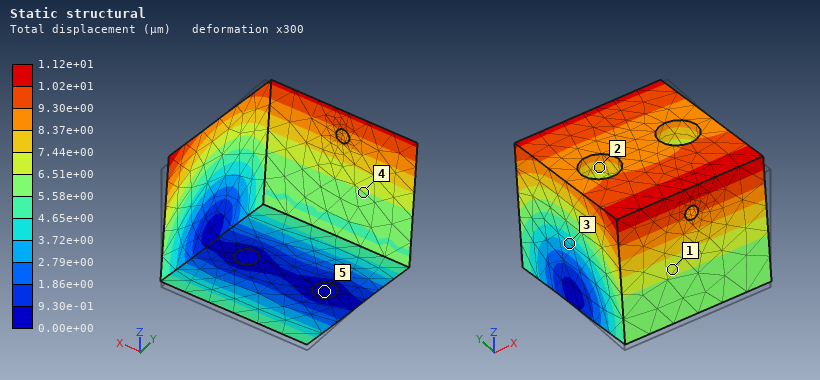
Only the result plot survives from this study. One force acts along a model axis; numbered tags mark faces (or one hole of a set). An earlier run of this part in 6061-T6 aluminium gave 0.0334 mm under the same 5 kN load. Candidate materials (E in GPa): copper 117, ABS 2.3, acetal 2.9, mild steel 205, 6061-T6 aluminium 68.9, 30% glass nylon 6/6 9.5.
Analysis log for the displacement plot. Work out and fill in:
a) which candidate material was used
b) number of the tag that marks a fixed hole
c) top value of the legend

mild steel
5
1.12e+01 µm
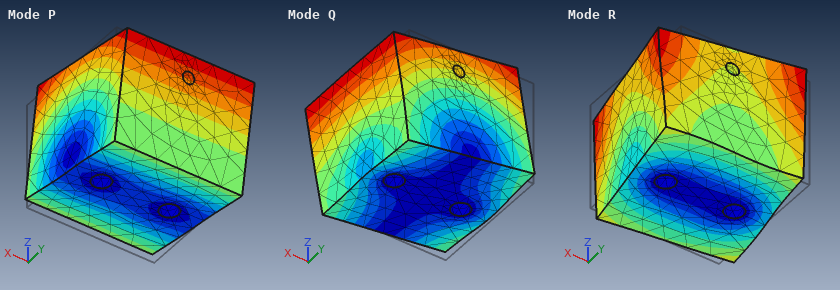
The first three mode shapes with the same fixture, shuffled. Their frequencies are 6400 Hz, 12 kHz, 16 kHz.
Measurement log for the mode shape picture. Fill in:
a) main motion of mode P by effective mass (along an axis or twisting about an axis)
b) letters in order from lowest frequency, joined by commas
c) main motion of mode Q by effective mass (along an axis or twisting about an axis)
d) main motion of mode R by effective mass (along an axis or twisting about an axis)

along Y
P, Q, R
along X
twisting about Z
